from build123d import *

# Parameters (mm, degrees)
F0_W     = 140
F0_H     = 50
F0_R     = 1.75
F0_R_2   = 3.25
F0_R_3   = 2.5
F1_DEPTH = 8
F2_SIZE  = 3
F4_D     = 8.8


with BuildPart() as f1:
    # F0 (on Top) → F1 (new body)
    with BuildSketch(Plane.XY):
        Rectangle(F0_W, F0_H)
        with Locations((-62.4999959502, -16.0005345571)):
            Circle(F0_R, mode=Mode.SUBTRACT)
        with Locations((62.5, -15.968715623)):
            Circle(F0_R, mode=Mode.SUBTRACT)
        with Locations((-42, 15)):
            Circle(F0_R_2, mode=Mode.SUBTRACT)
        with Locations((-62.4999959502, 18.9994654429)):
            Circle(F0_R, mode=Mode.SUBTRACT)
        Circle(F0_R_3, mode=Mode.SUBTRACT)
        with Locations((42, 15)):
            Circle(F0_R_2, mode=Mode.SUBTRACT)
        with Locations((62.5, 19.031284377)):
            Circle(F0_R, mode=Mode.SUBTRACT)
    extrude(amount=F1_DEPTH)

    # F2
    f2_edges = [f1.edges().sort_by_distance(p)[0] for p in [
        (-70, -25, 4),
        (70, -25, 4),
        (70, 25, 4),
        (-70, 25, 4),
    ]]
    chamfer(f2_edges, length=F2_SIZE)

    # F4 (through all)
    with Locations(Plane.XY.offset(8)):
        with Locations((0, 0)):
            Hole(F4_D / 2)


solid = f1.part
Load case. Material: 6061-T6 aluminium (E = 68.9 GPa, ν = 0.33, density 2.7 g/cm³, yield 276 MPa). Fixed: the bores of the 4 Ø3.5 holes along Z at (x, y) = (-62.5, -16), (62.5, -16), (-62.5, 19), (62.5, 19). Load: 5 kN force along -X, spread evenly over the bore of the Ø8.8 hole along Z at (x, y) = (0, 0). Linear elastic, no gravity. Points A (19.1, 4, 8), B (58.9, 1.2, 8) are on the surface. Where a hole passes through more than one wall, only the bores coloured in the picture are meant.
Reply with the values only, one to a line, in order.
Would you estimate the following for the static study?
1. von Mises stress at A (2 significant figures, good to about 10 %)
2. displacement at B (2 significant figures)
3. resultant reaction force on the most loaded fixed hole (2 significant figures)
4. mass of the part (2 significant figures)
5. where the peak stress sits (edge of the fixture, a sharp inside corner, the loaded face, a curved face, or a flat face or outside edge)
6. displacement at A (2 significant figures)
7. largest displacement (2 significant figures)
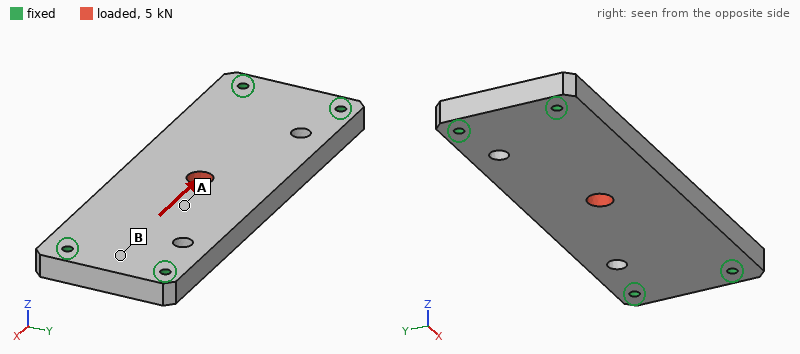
11 MPa
2.3 µm
1.4 kN
150 g
the loaded face
5.8 µm
9.3 µm
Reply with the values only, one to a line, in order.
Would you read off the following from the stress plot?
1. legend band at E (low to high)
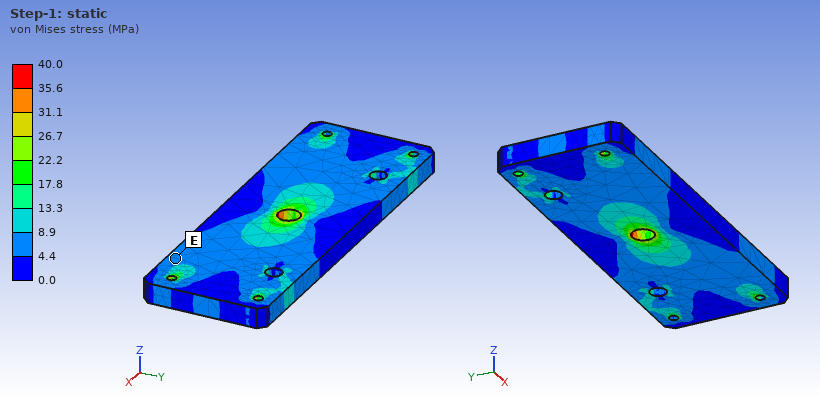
4.4 to 8.9 MPa
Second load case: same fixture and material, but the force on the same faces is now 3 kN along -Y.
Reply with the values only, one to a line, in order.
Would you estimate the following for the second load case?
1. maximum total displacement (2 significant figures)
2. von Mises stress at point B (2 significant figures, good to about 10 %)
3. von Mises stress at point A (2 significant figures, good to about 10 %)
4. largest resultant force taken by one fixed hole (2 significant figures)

18 µm
5.1 MPa
8.6 MPa
1.4 kN
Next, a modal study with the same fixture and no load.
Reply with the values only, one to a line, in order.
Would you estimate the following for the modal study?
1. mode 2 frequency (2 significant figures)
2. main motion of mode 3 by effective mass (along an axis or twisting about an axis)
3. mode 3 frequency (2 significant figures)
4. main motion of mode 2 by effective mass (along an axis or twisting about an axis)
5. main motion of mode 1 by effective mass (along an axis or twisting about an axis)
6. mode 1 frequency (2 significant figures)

4500 Hz
twisting about Y
6400 Hz
twisting about X
along Z
2400 Hz
